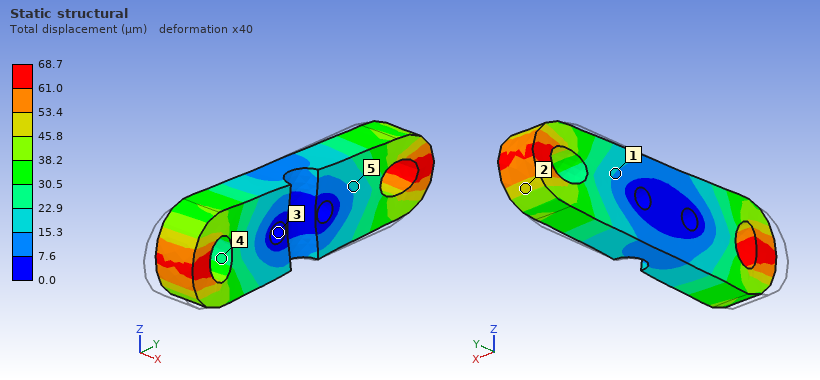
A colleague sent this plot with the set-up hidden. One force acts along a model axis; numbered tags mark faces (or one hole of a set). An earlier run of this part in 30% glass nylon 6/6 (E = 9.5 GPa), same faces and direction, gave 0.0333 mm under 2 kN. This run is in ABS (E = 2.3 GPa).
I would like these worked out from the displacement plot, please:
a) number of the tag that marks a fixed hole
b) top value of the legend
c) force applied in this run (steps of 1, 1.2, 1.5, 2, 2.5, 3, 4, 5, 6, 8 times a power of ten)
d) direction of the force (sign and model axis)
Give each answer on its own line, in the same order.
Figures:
3
68.7 µm
1 kN
+Y
